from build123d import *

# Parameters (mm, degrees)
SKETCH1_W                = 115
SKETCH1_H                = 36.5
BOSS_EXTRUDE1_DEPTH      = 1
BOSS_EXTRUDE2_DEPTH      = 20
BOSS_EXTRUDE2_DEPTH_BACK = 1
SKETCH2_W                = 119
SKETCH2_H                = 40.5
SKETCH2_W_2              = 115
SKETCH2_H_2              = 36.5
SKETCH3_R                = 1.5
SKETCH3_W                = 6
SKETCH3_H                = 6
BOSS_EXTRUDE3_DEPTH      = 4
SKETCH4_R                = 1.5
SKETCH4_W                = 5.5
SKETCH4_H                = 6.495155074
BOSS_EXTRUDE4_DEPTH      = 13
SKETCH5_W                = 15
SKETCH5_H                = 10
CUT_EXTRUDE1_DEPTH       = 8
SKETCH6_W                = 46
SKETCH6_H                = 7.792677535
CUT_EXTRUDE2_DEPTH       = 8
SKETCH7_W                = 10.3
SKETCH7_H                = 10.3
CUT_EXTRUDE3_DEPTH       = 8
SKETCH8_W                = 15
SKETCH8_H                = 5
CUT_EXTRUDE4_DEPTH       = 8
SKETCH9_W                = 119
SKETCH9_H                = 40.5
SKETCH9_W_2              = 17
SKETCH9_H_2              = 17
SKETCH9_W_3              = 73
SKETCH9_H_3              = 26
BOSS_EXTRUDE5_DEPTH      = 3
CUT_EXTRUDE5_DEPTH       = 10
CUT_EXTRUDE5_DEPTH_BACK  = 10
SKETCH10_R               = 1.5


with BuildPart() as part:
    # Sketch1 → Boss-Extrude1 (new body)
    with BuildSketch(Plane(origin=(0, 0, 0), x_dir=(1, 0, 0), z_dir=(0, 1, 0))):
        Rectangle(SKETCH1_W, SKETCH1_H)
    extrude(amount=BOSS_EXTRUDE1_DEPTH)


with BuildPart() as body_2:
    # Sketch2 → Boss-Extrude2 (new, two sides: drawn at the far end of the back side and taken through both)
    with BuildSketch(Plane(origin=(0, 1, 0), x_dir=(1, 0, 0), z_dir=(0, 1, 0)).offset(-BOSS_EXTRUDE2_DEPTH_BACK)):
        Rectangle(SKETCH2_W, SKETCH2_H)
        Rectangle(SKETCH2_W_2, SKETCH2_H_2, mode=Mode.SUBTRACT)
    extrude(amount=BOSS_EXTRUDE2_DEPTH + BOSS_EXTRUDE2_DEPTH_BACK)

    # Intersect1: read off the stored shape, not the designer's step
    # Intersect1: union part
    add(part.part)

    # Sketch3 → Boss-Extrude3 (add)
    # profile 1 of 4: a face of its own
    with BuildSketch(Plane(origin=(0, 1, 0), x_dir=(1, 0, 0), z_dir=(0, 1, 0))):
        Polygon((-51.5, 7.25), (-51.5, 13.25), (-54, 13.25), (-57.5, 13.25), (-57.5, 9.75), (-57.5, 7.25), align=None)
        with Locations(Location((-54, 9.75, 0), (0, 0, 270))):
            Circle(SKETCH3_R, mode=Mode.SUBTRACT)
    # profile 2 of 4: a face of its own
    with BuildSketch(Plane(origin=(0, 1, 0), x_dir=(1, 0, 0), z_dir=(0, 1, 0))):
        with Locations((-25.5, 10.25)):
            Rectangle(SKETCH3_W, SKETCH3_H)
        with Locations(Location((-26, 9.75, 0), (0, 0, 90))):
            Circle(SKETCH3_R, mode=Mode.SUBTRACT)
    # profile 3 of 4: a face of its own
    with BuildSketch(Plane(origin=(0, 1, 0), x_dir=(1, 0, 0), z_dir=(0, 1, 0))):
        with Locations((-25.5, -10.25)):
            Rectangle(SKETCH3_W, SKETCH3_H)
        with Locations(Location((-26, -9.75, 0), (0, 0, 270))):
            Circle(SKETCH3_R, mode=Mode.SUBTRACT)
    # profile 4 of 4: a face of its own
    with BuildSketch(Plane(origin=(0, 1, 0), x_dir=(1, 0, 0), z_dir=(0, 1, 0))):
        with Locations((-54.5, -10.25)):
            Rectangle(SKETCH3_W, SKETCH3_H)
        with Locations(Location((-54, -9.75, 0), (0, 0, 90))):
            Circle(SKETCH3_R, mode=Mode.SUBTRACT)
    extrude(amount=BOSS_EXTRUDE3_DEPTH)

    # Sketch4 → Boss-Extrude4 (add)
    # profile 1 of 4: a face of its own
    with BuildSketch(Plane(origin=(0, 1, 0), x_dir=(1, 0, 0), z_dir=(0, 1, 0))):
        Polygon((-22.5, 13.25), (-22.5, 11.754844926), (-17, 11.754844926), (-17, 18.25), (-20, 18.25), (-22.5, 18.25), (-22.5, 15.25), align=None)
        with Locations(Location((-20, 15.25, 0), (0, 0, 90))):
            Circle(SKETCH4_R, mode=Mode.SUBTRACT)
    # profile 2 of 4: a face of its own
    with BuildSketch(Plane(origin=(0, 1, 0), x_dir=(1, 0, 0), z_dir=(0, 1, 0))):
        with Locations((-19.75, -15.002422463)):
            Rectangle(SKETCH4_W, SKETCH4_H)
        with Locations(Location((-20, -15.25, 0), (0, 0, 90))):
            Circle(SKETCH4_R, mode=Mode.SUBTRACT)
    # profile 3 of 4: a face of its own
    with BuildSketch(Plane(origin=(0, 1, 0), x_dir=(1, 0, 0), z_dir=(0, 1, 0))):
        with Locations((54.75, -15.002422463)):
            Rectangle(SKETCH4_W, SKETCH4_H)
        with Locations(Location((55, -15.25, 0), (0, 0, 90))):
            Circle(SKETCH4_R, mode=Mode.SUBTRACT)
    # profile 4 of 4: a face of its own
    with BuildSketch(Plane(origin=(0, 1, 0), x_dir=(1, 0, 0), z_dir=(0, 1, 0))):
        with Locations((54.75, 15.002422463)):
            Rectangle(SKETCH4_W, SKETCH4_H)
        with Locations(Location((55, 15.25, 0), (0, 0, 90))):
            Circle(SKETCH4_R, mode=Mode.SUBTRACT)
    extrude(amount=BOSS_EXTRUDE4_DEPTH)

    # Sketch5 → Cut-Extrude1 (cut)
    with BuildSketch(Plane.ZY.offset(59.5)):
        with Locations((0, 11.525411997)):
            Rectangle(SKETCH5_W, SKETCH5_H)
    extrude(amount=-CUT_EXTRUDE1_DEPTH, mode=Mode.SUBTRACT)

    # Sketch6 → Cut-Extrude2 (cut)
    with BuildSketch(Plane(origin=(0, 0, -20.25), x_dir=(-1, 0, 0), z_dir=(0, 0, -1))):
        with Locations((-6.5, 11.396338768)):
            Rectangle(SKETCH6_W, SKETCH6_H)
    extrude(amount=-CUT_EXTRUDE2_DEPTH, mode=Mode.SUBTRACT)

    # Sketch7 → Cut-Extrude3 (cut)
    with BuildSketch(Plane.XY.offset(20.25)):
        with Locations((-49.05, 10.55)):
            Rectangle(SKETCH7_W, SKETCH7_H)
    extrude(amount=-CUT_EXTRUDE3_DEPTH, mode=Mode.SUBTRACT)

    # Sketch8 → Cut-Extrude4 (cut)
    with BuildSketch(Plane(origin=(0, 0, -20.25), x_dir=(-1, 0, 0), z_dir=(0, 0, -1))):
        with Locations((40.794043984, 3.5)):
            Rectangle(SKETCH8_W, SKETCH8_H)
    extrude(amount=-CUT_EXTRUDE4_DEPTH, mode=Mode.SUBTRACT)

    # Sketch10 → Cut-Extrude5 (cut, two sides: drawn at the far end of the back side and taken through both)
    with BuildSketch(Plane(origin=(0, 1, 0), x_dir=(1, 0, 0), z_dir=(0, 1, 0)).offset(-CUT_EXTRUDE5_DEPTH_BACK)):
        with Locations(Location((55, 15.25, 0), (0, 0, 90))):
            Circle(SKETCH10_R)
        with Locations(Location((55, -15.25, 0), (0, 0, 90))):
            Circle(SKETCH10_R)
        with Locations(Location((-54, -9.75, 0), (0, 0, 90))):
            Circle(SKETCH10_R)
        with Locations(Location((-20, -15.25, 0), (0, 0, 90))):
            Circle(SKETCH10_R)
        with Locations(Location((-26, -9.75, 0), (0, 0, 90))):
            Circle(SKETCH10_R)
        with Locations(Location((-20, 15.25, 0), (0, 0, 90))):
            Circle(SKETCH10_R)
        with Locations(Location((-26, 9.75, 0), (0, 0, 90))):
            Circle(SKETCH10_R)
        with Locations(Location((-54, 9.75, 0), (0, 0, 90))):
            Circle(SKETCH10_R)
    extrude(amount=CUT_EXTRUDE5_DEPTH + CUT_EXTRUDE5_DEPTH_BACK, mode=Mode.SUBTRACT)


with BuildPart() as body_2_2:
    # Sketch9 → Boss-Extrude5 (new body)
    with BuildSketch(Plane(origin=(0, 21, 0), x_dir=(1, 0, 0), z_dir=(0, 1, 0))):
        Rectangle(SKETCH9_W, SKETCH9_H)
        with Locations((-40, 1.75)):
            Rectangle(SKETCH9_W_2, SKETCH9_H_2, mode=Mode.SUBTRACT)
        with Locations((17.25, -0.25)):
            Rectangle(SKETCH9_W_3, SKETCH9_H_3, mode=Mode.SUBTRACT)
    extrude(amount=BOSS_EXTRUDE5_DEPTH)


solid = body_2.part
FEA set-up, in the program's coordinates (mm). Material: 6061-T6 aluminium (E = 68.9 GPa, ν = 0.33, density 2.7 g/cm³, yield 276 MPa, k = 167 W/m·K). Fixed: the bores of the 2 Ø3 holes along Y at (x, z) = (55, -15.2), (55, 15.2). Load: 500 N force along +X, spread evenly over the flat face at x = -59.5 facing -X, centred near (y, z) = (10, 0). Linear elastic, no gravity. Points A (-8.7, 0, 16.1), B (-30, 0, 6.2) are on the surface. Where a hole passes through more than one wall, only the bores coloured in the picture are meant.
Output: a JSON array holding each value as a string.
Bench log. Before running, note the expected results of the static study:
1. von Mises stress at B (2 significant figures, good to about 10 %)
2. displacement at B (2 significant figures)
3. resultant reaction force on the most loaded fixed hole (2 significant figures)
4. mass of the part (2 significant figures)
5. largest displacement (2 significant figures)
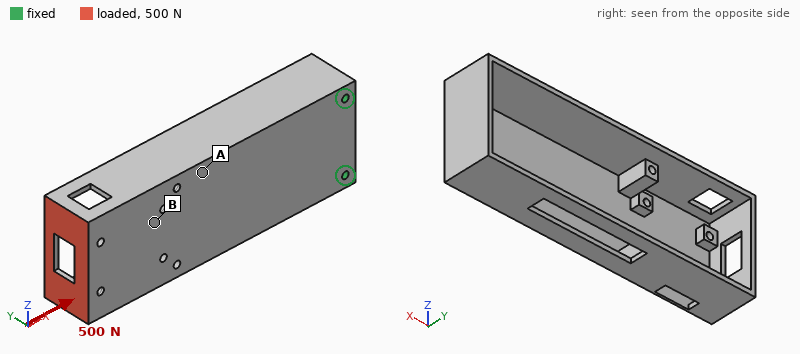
["9.3 MPa", "0.035 mm", "250 N", "48 g", "0.13 mm"]
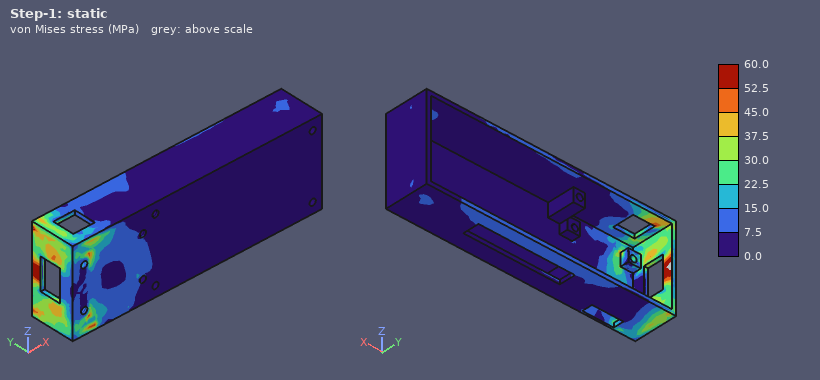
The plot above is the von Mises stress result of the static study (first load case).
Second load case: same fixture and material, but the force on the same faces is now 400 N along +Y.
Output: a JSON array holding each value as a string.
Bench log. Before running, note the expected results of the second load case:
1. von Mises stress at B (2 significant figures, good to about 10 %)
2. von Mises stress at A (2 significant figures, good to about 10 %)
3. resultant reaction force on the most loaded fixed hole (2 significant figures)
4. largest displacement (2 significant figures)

["18 MPa", "32 MPa", "210 N", "1.00 mm"]
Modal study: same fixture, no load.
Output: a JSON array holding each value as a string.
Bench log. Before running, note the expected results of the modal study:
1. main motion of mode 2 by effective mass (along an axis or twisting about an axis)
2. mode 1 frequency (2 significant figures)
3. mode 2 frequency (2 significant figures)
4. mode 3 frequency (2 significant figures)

["along Y", "760 Hz", "920 Hz", "1700 Hz"]
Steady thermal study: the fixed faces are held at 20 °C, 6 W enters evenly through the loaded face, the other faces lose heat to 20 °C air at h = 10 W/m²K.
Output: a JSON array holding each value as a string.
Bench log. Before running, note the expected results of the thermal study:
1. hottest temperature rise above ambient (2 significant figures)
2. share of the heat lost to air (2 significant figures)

["29 K", "42 %"]
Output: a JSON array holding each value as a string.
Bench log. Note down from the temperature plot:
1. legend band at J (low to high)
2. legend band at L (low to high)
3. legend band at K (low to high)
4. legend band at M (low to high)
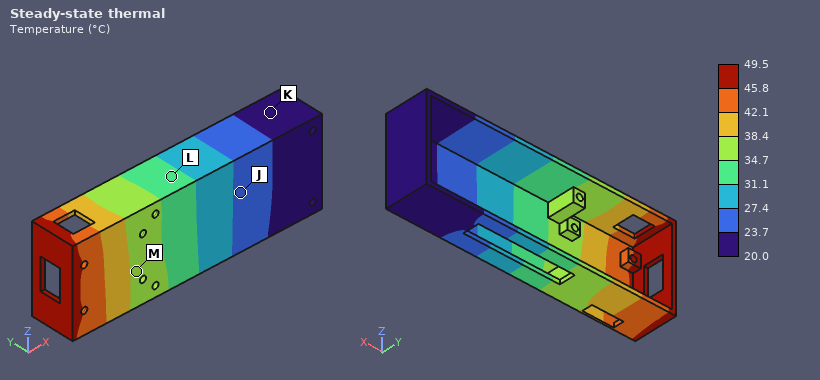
["23.7 to 27.4 °C", "31.1 to 34.7 °C", "20.0 to 23.7 °C", "34.7 to 38.4 °C"]
